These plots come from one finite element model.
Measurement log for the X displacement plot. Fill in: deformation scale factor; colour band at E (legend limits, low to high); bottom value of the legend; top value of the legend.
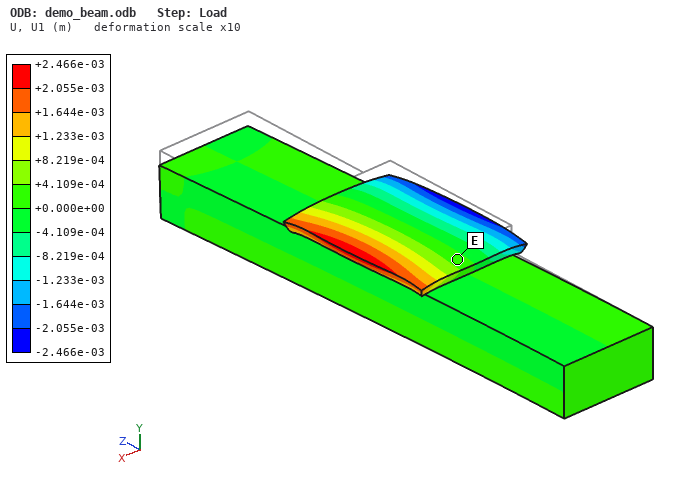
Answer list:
10
+0.000e+00 to +4.109e-04 m
-2.466e-03 m
+2.466e-03 m
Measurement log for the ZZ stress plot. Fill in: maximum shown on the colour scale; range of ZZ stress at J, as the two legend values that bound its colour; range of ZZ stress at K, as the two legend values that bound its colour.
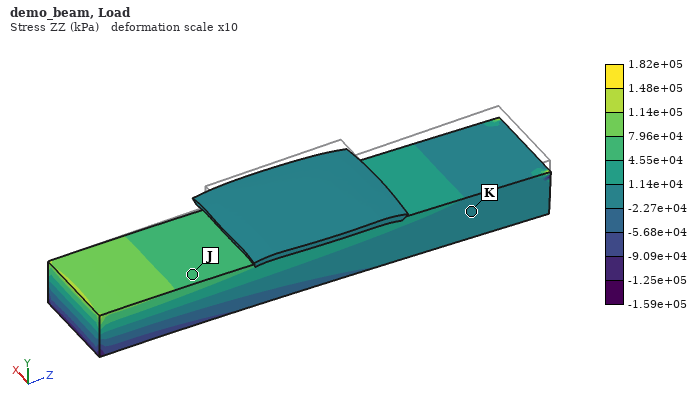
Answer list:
1.82e+05 kPa
4.55e+04 to 7.96e+04 kPa
-2.27e+04 to 1.14e+04 kPa
